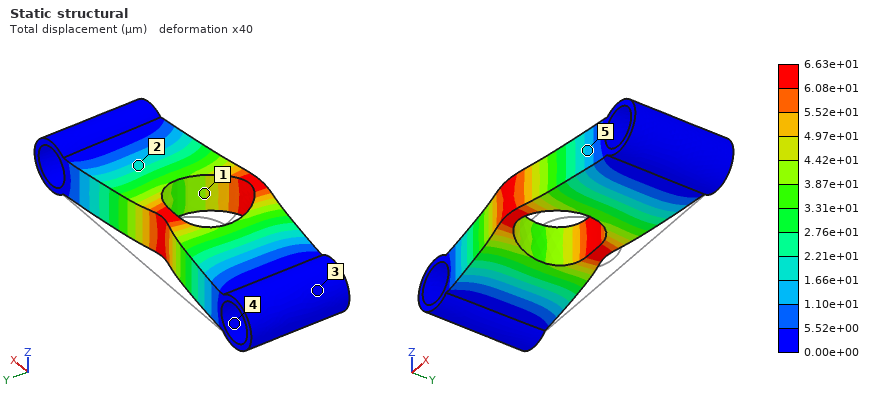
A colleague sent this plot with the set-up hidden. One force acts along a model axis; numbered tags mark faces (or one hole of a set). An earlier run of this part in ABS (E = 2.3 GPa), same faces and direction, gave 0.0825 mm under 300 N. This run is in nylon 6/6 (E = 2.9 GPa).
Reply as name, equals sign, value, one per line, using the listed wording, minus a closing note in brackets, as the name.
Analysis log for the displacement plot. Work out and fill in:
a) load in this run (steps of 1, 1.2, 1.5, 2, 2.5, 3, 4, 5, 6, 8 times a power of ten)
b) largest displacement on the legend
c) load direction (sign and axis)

load in this run = 300 N
largest displacement on the legend = 6.63e+01 µm
load direction = -Y
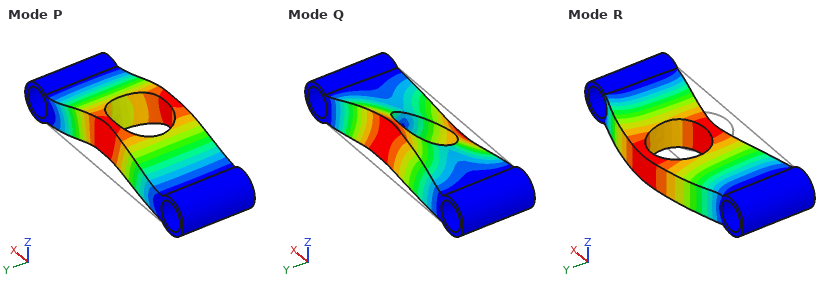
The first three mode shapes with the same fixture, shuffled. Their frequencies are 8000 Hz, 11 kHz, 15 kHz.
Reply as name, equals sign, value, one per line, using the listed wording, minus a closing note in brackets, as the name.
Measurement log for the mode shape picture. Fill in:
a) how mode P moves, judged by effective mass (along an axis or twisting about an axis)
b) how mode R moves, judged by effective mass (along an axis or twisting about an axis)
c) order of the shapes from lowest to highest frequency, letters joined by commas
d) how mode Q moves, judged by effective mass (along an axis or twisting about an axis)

how mode P moves, judged by effective mass = along Z
how mode R moves, judged by effective mass = along Y
order of the shapes from lowest to highest frequency, letters joined by commas = P, Q, R
how mode Q moves, judged by effective mass = twisting about X
